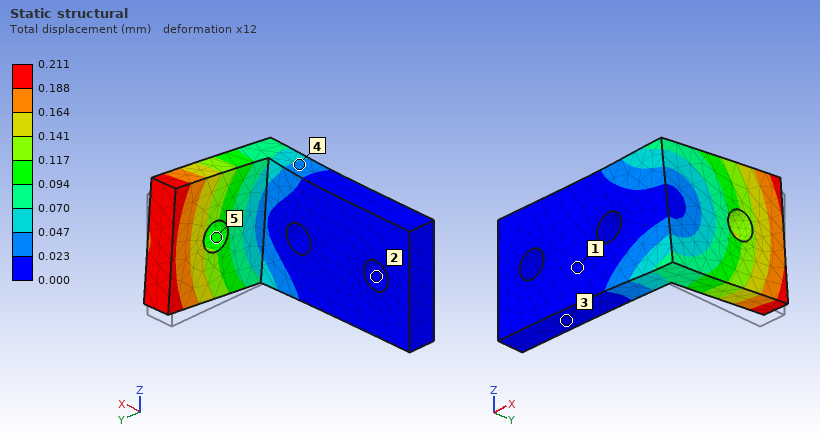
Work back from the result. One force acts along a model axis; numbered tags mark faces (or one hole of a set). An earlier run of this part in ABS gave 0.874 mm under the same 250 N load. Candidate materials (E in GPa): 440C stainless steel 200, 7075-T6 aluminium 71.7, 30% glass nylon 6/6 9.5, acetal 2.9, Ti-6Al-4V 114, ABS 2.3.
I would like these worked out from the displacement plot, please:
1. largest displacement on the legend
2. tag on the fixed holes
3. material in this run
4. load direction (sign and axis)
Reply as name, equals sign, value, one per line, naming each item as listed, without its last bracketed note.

largest displacement on the legend = 0.211 mm
tag on the fixed holes = 2
material in this run = 30% glass nylon 6/6
load direction = +Z
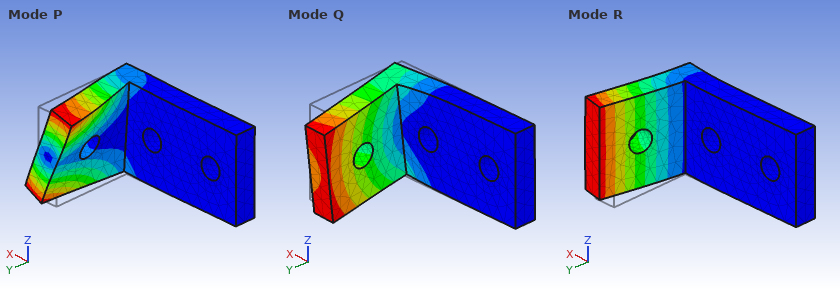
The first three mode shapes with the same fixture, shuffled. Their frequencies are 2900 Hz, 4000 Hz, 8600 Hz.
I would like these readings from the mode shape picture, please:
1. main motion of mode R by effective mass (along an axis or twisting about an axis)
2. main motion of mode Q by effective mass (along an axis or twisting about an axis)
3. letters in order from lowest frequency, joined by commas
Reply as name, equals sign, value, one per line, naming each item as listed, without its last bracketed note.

main motion of mode R by effective mass = along X
main motion of mode Q by effective mass = along Z
letters in order from lowest frequency, joined by commas = R, Q, P
